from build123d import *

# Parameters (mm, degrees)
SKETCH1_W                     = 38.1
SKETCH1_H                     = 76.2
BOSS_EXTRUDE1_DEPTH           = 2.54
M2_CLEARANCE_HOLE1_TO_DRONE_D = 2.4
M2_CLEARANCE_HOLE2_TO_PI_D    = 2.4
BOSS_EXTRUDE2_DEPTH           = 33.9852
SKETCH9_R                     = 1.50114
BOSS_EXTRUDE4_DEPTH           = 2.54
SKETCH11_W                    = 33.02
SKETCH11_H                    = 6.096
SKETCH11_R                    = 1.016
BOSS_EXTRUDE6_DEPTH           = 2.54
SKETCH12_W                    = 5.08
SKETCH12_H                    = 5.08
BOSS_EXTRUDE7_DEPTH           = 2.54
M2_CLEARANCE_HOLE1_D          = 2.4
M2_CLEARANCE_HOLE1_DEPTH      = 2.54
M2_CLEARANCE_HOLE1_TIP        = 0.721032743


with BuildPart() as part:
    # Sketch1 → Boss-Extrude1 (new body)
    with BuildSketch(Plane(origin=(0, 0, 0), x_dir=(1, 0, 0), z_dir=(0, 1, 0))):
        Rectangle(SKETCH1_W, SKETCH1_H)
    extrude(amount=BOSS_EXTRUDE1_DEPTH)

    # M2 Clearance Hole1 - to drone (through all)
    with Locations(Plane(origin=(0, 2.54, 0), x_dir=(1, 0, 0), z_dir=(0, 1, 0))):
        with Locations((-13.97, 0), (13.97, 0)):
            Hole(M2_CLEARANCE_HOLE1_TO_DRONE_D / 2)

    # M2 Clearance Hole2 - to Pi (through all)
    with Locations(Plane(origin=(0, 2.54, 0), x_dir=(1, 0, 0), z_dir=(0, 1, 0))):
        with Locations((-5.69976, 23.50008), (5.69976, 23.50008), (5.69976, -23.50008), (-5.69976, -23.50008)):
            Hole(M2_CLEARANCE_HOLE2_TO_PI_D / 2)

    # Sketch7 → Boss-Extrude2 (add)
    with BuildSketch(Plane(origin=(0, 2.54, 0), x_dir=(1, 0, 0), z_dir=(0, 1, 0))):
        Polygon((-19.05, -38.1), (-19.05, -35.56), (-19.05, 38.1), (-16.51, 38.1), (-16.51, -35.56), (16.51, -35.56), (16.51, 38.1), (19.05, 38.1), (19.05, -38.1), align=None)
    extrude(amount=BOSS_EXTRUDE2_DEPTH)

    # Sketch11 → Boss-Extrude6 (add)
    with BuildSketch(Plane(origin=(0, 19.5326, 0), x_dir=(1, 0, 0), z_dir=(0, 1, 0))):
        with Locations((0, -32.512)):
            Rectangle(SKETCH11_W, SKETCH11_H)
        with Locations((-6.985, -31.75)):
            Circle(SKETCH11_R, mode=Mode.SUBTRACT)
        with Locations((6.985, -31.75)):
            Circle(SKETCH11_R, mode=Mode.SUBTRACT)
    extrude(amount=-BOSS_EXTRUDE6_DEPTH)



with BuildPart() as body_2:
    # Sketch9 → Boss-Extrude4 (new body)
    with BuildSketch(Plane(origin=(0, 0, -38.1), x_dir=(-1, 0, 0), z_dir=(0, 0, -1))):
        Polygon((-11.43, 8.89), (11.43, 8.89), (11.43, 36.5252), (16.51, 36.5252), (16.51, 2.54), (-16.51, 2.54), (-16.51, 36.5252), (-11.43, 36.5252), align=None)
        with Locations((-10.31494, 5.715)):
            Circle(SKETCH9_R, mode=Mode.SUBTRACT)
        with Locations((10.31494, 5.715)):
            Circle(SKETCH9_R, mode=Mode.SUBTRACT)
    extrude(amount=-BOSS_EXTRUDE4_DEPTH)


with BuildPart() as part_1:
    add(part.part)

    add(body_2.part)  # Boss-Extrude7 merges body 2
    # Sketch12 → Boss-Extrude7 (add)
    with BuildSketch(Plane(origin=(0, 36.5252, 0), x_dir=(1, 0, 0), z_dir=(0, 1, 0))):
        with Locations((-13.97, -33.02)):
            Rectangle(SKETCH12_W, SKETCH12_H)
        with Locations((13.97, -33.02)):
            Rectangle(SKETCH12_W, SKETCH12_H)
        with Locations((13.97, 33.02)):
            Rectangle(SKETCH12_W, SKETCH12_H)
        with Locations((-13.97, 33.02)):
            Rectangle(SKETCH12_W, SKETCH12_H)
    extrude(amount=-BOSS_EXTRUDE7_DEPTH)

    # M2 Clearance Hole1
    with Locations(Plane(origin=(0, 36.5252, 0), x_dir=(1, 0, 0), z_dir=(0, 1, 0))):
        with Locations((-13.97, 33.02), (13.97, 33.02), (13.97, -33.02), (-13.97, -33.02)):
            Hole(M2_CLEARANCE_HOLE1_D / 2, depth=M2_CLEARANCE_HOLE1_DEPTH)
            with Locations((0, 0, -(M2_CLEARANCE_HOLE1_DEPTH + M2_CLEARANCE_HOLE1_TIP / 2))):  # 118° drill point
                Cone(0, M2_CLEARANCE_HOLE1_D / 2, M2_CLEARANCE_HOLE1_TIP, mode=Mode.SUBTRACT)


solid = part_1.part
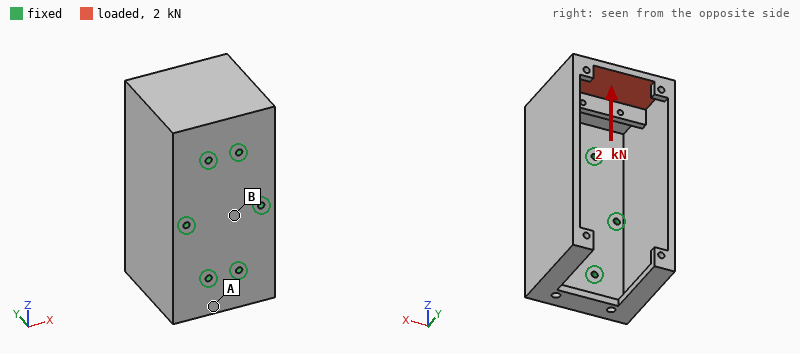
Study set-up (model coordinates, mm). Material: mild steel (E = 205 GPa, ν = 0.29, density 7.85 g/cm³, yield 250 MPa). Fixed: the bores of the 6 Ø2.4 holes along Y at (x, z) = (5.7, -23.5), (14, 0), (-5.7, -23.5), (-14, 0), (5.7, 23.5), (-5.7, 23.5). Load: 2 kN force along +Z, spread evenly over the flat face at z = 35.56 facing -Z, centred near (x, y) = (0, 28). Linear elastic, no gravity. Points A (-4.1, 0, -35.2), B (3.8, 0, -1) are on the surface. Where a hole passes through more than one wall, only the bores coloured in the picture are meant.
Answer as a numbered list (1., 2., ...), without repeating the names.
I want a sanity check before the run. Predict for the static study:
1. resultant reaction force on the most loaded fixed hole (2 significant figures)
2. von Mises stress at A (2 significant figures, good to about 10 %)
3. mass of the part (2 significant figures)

1. 660 N
2. 47 MPa
3. 200 g
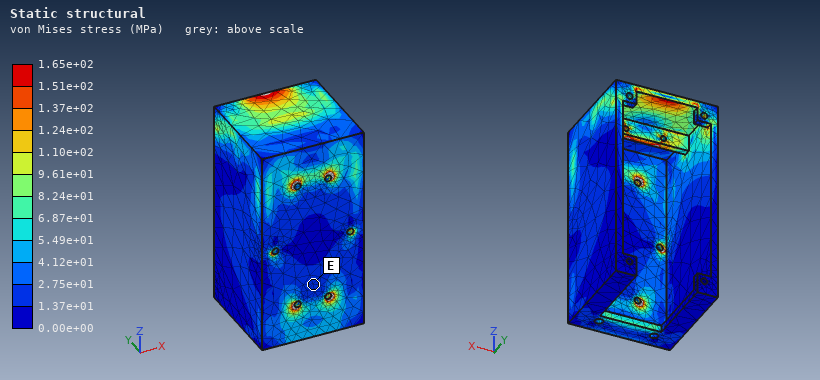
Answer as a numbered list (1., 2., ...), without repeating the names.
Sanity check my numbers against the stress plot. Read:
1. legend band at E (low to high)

1. 1.37e+01 to 2.75e+01 MPa
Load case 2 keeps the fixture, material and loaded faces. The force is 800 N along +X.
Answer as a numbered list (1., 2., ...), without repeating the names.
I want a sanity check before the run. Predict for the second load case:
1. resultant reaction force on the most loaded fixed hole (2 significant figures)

1. 790 N
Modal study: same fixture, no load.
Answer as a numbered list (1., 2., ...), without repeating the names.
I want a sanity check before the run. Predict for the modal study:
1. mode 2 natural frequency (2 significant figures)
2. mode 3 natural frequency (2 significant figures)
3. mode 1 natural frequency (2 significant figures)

1. 2300 Hz
2. 2400 Hz
3. 2000 Hz
